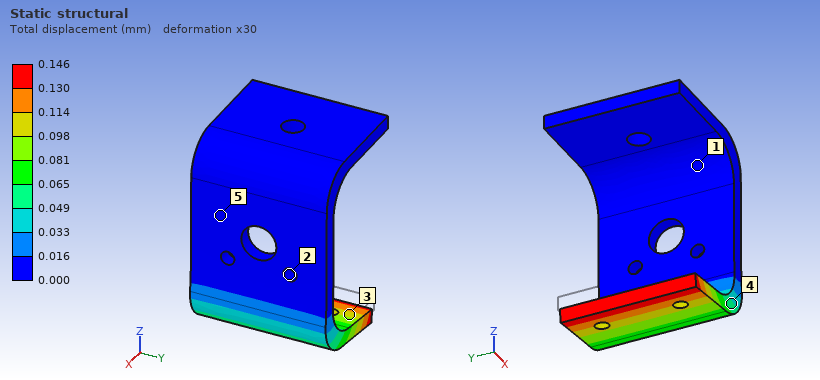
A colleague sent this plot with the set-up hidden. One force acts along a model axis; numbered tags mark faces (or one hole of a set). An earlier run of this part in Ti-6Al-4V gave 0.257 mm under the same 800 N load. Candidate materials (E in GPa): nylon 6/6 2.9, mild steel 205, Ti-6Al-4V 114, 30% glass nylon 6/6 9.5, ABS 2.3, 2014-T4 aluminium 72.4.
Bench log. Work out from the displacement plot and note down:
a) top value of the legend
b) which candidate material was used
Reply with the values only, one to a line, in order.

0.146 mm
mild steel
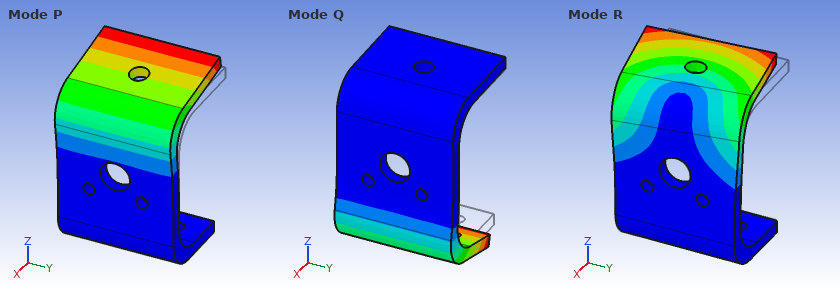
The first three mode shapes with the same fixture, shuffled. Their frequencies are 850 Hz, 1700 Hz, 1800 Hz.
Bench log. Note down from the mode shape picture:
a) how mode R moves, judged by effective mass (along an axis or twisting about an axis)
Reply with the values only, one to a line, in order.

along Y
